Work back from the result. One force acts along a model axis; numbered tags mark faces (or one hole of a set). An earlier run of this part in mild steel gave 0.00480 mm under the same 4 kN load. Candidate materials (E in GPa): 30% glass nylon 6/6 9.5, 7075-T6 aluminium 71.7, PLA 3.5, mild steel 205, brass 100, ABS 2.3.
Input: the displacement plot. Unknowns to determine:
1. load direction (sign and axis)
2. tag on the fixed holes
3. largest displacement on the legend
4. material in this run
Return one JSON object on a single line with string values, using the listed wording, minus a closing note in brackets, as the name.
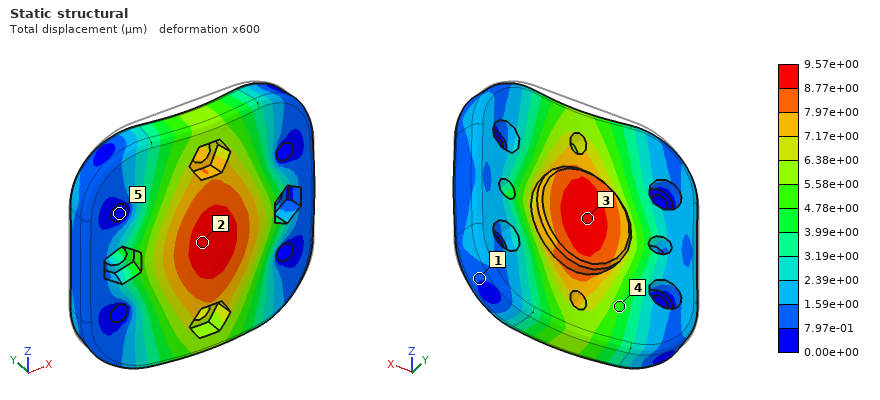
{"load direction": "-Y", "tag on the fixed holes": "5", "largest displacement on the legend": "9.57e+00 µm", "material in this run": "brass"}
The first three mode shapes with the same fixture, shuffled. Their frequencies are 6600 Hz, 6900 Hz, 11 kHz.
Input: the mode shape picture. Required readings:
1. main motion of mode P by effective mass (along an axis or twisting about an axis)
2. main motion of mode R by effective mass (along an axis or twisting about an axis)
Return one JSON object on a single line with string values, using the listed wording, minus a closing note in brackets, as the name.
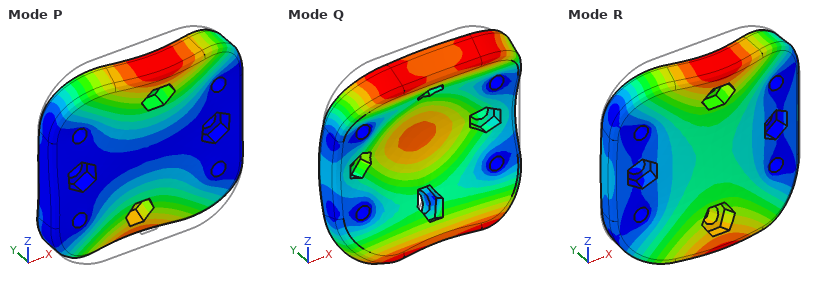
{"main motion of mode P by effective mass": "twisting about X", "main motion of mode R by effective mass": "along Y"}
